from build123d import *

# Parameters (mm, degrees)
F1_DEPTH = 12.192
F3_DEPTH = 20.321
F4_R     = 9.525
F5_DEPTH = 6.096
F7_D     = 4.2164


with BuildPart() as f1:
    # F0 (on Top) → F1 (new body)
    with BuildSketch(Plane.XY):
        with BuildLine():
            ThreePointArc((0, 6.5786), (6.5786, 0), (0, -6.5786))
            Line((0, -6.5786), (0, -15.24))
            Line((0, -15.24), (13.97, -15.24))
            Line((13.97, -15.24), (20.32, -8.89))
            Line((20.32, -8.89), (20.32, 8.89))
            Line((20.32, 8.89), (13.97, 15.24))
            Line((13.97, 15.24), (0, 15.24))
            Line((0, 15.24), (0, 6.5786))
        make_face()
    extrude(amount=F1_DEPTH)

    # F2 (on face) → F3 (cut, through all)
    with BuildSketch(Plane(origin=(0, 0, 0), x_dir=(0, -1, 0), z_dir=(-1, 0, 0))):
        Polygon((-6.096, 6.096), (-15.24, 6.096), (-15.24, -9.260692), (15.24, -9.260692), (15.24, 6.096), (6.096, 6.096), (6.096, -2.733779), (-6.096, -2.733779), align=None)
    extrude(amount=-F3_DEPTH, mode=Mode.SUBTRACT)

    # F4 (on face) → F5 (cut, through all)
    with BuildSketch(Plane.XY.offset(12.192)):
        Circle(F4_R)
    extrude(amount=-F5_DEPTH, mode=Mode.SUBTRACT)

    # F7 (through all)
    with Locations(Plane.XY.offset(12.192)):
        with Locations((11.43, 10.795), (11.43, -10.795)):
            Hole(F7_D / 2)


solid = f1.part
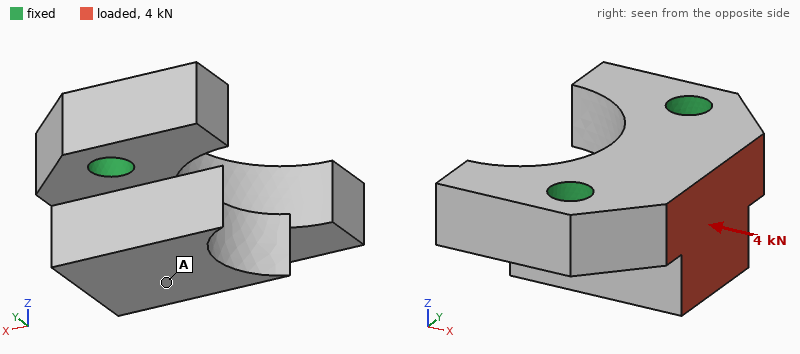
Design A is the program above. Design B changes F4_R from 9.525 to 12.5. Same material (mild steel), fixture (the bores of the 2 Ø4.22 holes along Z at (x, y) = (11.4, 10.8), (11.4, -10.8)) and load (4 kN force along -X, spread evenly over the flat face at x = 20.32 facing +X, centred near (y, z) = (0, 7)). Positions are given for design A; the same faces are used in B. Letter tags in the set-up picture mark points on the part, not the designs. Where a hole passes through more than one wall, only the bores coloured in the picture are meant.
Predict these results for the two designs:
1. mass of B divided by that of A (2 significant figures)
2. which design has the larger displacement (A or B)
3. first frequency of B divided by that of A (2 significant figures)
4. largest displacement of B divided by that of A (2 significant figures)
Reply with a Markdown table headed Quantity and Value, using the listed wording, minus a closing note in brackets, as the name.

| Quantity | Value |
|---|---|
| mass of B divided by that of A | 0.83 |
| which design has the larger displacement | B |
| first frequency of B divided by that of A | 0.76 |
| largest displacement of B divided by that of A | 1.9 |
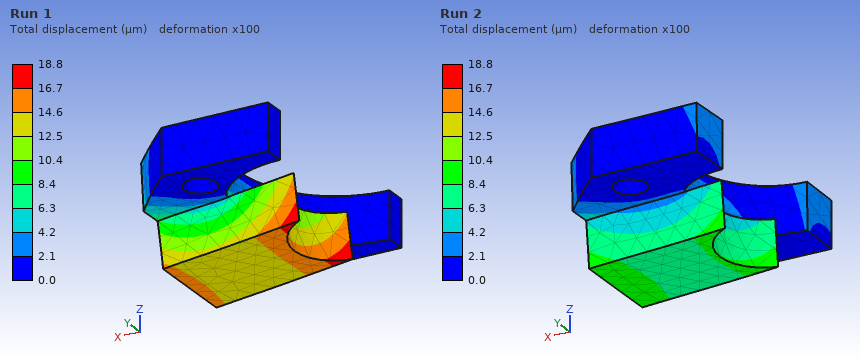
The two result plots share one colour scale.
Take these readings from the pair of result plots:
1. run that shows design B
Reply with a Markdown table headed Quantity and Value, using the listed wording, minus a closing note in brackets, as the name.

| Quantity | Value |
|---|---|
| run that shows design B | Run 1 |
